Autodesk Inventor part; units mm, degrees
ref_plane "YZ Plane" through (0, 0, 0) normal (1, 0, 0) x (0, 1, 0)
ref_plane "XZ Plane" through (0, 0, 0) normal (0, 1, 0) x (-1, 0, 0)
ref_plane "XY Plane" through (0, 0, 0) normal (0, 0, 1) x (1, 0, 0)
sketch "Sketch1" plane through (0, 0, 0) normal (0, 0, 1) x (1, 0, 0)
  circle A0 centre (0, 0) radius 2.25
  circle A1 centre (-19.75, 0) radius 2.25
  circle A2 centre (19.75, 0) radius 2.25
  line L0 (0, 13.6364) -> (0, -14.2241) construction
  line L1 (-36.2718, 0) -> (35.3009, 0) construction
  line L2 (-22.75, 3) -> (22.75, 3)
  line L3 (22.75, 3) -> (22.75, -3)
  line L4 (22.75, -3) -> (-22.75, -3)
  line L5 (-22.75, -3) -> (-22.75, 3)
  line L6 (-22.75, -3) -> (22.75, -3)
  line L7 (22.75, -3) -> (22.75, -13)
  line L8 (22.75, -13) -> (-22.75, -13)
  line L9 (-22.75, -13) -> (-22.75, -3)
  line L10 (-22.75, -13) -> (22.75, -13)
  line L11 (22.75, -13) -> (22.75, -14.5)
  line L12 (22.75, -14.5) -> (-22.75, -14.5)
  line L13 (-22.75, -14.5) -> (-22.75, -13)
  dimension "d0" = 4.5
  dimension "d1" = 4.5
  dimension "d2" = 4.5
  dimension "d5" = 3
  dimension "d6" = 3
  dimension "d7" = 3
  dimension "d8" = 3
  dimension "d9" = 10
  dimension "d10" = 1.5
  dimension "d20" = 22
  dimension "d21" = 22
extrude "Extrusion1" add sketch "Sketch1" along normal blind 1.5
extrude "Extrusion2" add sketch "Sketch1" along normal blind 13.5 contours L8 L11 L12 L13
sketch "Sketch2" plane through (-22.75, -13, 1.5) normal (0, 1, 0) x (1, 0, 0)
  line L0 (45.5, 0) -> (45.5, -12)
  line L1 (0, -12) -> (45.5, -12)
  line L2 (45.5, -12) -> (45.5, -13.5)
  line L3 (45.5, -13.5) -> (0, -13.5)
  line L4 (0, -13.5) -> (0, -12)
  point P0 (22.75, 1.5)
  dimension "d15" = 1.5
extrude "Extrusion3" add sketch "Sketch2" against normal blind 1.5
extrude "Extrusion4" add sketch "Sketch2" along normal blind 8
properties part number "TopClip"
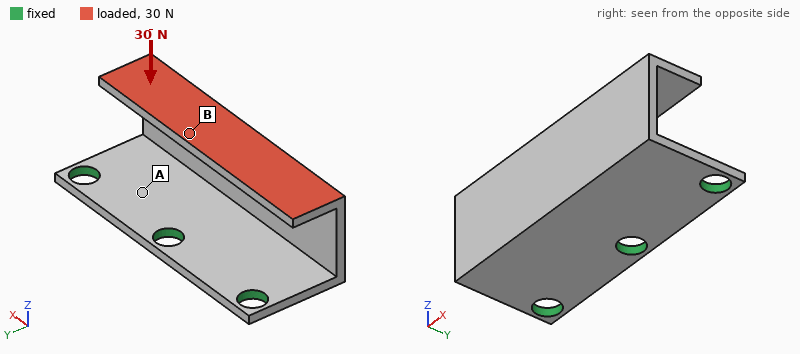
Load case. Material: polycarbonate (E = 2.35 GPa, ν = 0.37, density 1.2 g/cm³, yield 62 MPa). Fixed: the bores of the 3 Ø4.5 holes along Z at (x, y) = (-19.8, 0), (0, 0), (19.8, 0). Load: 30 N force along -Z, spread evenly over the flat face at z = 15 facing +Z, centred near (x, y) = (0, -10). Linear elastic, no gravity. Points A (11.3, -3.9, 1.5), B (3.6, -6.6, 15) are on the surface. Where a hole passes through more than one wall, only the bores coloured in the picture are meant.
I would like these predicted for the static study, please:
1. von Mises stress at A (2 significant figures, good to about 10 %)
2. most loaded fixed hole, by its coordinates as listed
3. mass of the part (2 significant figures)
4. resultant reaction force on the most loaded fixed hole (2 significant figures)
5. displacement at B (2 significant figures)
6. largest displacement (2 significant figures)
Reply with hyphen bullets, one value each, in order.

- 5.3 MPa
- (0, 0)
- 3.1 g
- 13 N
- 0.52 mm
- 0.58 mm
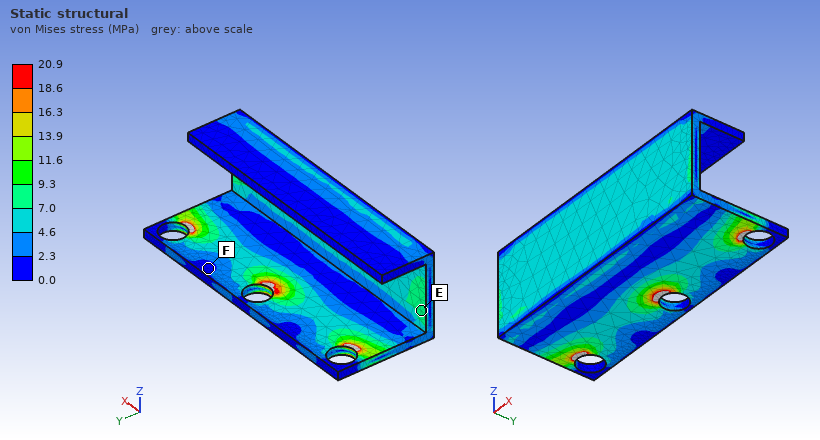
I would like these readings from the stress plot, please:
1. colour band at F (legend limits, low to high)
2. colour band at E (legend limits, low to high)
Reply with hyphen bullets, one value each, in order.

- 0.0 to 2.3 MPa
- 7.0 to 9.3 MPa
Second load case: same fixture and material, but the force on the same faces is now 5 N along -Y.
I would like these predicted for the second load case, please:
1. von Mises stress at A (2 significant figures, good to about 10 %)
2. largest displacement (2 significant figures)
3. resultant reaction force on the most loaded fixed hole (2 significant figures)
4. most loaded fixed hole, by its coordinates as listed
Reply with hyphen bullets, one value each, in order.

- 2.7 MPa
- 0.56 mm
- 2.6 N
- (0, 0)
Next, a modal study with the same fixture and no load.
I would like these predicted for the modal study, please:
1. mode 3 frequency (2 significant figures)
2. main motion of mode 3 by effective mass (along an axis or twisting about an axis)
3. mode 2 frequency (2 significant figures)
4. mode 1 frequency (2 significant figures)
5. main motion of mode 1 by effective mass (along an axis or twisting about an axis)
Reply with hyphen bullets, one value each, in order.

- 1100 Hz
- along Z
- 740 Hz
- 460 Hz
- along Y
